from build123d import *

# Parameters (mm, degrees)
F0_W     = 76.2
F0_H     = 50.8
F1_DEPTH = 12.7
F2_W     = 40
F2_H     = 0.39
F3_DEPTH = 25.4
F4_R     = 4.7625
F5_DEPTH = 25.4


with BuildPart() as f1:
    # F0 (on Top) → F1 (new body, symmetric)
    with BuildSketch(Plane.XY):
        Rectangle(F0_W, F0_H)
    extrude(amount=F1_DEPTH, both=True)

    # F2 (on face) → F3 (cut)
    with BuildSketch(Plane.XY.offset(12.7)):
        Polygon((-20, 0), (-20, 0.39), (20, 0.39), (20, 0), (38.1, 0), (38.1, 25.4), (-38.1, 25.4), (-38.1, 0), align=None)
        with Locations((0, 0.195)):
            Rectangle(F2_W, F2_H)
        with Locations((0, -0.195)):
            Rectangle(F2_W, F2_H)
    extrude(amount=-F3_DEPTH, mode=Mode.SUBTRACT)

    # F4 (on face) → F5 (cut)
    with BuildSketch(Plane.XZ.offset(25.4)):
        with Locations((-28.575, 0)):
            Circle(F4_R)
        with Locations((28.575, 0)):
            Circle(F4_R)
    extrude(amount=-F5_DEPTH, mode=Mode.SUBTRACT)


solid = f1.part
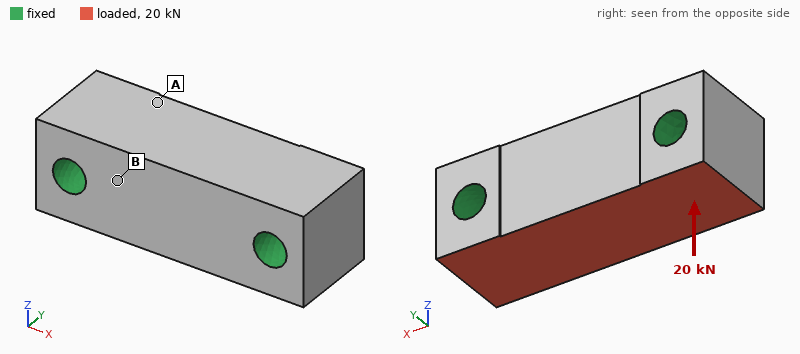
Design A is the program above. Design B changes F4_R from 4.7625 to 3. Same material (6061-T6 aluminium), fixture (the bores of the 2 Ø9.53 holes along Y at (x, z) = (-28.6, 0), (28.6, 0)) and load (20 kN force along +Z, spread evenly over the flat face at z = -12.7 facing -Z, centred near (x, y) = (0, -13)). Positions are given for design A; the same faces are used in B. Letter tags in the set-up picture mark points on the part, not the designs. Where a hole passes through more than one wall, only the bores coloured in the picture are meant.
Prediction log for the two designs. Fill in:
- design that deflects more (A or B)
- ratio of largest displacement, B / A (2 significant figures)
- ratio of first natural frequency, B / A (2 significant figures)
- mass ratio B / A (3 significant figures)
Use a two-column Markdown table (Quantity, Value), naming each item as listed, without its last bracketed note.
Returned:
| Quantity | Value |
|---|---|
| design that deflects more | B |
| ratio of largest displacement, B / A | 1.3 |
| ratio of first natural frequency, B / A | 0.83 |
| mass ratio B / A | 1.05 |
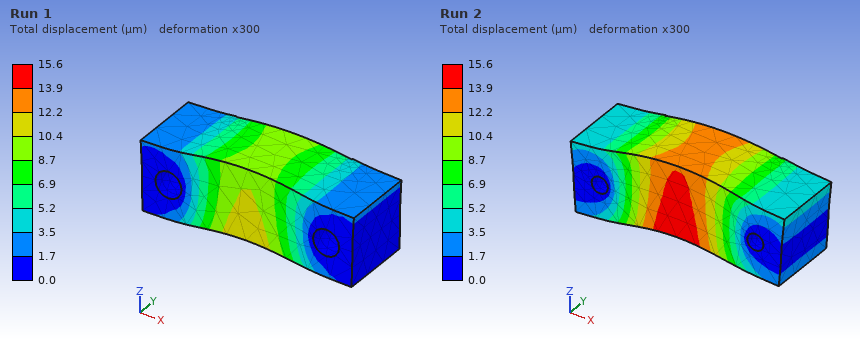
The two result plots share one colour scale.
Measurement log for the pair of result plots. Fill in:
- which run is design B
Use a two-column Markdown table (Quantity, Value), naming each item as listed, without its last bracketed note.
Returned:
| Quantity | Value |
|---|---|
| which run is design B | Run 2 |
